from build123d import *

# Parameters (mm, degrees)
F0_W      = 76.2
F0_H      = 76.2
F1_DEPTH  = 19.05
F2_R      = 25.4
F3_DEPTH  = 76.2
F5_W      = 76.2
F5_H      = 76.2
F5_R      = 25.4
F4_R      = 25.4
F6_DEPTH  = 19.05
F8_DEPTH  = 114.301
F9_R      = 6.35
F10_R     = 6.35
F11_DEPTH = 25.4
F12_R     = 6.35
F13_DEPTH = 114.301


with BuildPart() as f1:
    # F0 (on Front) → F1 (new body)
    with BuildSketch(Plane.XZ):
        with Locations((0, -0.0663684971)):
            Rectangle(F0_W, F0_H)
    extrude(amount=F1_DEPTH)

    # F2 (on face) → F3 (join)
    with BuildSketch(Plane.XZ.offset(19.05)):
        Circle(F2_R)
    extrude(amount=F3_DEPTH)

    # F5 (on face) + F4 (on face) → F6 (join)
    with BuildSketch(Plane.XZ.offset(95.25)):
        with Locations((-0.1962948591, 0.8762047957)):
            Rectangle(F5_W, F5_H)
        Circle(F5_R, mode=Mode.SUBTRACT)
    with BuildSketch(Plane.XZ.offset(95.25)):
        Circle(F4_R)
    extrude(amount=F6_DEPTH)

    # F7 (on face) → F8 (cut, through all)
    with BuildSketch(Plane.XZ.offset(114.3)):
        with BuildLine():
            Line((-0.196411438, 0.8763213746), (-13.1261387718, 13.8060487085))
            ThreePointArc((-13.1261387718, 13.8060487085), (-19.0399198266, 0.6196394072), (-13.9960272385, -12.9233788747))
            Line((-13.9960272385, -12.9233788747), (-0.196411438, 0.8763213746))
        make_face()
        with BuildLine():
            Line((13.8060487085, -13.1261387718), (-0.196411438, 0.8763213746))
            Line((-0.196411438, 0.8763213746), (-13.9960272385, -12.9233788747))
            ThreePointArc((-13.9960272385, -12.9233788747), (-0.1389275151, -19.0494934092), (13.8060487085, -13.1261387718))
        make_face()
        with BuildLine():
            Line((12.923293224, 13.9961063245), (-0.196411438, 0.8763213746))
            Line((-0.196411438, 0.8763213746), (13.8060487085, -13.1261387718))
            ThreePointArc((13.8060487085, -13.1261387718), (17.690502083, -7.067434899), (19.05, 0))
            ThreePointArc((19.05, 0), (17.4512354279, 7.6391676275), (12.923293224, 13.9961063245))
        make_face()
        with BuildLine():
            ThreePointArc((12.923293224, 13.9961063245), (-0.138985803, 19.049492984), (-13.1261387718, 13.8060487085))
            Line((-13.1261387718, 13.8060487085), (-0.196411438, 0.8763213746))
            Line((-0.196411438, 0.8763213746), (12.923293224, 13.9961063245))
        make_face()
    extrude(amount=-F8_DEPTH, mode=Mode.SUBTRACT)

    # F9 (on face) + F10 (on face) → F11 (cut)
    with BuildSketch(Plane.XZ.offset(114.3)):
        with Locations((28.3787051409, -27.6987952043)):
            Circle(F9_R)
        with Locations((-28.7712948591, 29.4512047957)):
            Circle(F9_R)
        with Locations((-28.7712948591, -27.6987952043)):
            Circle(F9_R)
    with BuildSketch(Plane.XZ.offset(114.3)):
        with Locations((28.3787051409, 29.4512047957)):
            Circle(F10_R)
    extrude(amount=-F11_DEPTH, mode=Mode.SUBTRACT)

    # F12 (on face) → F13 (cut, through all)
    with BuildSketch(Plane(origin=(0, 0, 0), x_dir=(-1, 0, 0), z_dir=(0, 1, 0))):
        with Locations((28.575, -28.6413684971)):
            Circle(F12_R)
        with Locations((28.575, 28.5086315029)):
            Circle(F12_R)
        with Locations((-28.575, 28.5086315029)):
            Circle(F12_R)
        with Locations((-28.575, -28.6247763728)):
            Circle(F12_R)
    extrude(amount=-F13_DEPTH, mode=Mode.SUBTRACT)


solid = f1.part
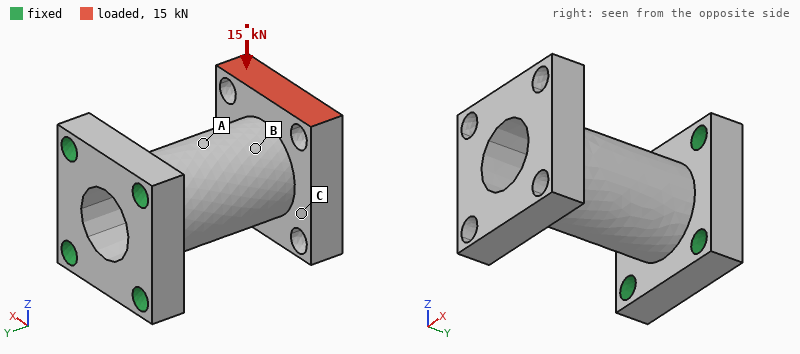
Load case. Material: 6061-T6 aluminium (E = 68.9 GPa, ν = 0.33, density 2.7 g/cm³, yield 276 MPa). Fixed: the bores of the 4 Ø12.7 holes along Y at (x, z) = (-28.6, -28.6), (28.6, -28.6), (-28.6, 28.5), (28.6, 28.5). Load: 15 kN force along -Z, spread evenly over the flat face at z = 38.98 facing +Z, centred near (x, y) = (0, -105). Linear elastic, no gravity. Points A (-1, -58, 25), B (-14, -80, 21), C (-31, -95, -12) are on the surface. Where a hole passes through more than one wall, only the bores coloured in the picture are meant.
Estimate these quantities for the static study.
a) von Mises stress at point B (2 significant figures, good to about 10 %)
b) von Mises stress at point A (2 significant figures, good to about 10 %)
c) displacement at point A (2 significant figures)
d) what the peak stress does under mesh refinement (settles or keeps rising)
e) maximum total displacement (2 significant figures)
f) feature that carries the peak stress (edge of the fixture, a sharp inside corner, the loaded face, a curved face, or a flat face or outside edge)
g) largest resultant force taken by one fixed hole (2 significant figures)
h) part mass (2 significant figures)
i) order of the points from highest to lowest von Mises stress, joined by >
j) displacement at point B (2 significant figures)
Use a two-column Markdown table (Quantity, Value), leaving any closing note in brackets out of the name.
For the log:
| Quantity | Value |
|---|---|
| von Mises stress at point B | 46 MPa |
| von Mises stress at point A | 83 MPa |
| displacement at point A | 0.20 mm |
| what the peak stress does under mesh refinement | keeps rising |
| maximum total displacement | 0.54 mm |
| feature that carries the peak stress | edge of the fixture |
| largest resultant force taken by one fixed hole | 15 kN |
| part mass | 610 g |
| order of the points from highest to lowest von Mises stress, joined by > | A > B > C |
| displacement at point B | 0.31 mm |
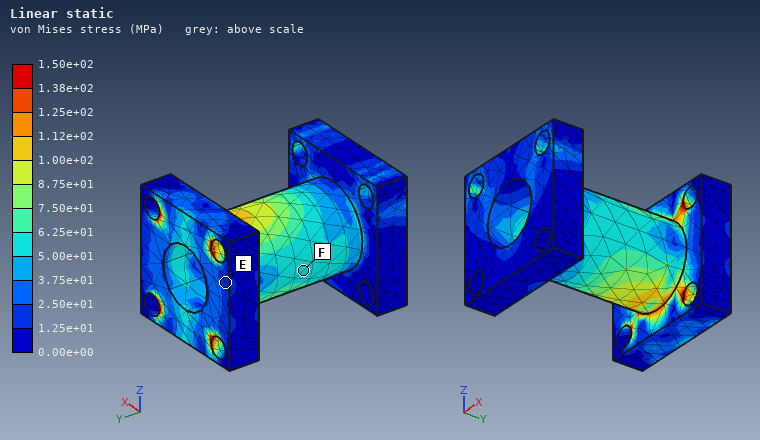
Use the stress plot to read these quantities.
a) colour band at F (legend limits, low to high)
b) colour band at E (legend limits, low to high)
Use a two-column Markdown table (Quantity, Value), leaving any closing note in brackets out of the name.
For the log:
| Quantity | Value |
|---|---|
| colour band at F | 5.00e+01 to 6.25e+01 MPa |
| colour band at E | 1.25e+01 to 2.50e+01 MPa |
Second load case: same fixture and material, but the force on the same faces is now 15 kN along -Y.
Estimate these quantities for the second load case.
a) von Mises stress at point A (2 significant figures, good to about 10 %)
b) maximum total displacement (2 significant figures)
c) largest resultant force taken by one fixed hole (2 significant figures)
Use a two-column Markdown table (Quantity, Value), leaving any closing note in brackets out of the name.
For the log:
| Quantity | Value |
|---|---|
| von Mises stress at point A | 85 MPa |
| maximum total displacement | 0.39 mm |
| largest resultant force taken by one fixed hole | 10 kN |
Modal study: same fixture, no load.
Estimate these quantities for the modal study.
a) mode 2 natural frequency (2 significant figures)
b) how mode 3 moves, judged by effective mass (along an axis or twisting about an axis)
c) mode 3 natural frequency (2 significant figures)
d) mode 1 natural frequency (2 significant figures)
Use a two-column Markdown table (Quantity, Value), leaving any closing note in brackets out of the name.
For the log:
| Quantity | Value |
|---|---|
| mode 2 natural frequency | 1800 Hz |
| how mode 3 moves, judged by effective mass | twisting about Y |
| mode 3 natural frequency | 3600 Hz |
| mode 1 natural frequency | 1800 Hz |
